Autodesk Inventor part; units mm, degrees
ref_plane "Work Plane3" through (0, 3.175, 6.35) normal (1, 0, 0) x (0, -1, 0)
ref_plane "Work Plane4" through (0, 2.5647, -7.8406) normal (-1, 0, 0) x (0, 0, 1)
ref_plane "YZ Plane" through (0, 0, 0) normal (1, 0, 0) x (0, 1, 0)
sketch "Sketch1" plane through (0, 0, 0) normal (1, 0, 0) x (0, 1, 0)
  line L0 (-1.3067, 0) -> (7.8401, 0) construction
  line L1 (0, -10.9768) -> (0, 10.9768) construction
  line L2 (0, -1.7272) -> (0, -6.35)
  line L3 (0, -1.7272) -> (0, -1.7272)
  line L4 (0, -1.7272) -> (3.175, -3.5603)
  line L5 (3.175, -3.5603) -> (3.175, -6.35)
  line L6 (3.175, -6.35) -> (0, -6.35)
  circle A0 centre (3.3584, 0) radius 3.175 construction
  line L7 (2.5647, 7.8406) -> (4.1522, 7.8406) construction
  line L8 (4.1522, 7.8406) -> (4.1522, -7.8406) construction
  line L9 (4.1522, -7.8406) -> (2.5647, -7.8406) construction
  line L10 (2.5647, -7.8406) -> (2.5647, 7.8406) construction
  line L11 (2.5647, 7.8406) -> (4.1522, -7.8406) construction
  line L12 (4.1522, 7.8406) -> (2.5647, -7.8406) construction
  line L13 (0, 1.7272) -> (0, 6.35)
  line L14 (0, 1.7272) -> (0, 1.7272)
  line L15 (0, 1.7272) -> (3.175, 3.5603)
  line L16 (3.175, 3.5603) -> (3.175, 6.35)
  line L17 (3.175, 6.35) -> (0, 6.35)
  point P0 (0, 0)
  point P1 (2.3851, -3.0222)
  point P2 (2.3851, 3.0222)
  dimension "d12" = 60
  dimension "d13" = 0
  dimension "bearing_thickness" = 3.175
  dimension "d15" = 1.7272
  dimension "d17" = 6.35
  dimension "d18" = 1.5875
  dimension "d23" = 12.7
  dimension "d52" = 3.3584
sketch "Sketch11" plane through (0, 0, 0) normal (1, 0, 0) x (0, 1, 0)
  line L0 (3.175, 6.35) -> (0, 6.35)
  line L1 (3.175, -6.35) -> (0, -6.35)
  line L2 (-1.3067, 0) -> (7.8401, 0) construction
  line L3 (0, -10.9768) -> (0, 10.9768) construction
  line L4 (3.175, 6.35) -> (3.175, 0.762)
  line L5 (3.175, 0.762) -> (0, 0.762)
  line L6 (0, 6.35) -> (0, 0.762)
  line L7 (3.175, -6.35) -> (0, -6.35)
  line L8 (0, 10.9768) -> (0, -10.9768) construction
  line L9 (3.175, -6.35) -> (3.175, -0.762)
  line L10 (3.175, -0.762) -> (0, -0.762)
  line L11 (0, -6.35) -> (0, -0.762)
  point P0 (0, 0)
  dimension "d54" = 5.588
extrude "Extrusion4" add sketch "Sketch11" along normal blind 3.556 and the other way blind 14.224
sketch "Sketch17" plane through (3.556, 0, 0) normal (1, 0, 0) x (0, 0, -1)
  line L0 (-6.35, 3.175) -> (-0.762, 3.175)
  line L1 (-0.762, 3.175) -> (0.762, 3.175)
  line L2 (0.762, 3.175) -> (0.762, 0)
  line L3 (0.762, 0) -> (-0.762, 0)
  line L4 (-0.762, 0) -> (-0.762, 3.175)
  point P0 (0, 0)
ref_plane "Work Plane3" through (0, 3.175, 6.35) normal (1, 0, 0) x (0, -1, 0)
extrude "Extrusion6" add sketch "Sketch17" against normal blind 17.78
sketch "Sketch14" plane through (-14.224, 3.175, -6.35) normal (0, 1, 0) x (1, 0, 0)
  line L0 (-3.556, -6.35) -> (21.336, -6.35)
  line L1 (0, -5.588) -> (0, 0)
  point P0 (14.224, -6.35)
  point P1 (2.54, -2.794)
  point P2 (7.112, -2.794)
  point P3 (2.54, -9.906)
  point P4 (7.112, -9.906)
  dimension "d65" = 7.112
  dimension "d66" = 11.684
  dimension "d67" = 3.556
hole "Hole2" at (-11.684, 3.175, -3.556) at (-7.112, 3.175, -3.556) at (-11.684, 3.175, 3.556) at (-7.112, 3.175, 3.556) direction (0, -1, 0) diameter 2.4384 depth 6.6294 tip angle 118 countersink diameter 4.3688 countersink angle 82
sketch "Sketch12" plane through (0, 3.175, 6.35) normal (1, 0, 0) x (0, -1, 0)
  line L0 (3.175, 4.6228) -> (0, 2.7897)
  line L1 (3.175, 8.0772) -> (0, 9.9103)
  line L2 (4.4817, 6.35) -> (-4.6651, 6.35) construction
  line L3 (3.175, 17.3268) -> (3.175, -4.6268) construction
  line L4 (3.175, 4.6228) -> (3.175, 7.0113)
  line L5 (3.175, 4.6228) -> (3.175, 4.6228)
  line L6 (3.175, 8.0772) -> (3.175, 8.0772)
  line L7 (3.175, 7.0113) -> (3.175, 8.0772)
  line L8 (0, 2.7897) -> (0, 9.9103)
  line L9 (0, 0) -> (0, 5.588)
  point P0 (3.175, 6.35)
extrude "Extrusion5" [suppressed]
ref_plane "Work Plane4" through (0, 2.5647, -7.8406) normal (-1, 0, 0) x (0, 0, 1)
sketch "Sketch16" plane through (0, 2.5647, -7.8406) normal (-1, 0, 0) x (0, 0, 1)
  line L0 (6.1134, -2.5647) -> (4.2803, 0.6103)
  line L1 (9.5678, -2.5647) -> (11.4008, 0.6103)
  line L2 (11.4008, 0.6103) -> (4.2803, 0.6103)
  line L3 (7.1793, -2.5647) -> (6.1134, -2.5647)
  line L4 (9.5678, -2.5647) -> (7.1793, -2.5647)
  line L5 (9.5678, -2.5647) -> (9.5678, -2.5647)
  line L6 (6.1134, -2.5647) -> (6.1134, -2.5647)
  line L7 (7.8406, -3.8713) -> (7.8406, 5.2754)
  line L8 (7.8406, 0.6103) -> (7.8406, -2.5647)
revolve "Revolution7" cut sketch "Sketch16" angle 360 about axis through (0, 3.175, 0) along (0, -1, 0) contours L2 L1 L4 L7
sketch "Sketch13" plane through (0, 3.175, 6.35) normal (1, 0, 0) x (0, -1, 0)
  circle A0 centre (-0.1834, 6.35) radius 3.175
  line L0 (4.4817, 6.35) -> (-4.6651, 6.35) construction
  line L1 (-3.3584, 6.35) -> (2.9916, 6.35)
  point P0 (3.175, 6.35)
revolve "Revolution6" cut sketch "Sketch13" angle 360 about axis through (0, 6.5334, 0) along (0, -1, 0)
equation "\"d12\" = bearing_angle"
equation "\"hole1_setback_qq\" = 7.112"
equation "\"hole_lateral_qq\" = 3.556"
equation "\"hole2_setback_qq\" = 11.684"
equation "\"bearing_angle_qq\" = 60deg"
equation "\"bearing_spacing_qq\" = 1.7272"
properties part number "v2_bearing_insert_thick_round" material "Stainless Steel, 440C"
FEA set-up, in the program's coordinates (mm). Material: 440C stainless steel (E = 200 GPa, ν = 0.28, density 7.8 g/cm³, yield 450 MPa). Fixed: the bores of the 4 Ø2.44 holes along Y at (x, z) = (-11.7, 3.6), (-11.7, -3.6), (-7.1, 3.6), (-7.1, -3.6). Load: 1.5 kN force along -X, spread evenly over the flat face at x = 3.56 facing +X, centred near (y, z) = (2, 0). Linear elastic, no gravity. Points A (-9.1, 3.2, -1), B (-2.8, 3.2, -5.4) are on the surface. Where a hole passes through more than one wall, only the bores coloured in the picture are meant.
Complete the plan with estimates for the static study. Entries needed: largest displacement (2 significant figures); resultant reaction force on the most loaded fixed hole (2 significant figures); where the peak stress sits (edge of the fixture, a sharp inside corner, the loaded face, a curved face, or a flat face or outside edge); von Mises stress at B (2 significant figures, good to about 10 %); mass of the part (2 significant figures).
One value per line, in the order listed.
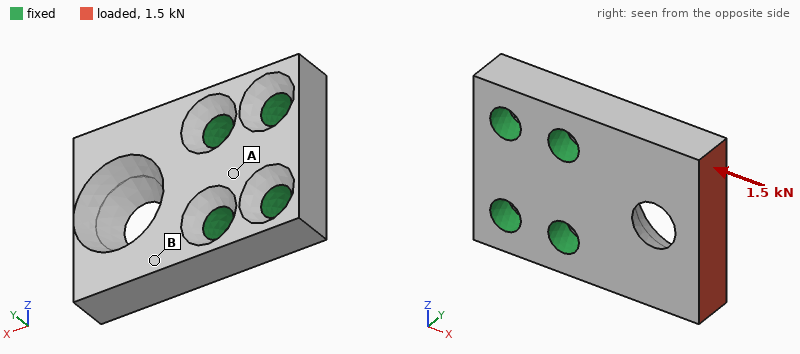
19 µm
660 N
the loaded face
65 MPa
4.4 g
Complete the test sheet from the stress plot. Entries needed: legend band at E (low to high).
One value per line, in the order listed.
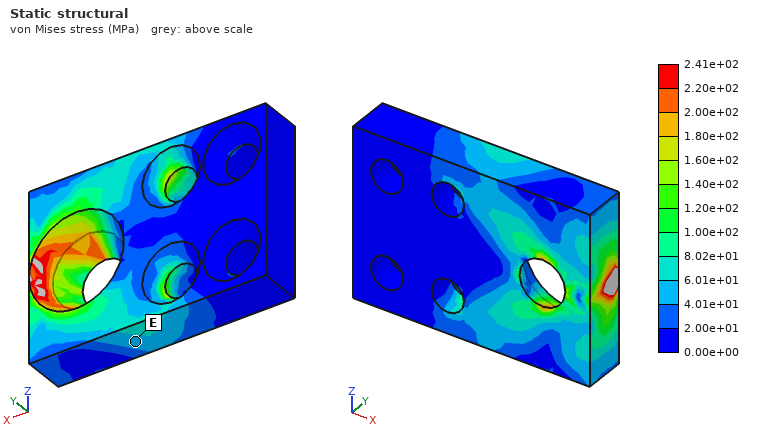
4.01e+01 to 6.01e+01 MPa
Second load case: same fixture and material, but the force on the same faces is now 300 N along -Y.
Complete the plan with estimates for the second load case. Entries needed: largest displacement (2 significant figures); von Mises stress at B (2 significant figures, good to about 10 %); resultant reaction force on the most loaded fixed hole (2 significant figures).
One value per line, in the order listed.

29 µm
130 MPa
250 N
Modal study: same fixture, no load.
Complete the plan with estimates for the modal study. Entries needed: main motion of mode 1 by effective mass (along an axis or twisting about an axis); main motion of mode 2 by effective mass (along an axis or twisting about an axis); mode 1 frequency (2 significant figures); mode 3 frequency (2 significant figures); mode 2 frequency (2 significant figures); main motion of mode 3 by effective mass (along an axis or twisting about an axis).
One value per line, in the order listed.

along Y
twisting about X
21 kHz
46 kHz
34 kHz
along Z
